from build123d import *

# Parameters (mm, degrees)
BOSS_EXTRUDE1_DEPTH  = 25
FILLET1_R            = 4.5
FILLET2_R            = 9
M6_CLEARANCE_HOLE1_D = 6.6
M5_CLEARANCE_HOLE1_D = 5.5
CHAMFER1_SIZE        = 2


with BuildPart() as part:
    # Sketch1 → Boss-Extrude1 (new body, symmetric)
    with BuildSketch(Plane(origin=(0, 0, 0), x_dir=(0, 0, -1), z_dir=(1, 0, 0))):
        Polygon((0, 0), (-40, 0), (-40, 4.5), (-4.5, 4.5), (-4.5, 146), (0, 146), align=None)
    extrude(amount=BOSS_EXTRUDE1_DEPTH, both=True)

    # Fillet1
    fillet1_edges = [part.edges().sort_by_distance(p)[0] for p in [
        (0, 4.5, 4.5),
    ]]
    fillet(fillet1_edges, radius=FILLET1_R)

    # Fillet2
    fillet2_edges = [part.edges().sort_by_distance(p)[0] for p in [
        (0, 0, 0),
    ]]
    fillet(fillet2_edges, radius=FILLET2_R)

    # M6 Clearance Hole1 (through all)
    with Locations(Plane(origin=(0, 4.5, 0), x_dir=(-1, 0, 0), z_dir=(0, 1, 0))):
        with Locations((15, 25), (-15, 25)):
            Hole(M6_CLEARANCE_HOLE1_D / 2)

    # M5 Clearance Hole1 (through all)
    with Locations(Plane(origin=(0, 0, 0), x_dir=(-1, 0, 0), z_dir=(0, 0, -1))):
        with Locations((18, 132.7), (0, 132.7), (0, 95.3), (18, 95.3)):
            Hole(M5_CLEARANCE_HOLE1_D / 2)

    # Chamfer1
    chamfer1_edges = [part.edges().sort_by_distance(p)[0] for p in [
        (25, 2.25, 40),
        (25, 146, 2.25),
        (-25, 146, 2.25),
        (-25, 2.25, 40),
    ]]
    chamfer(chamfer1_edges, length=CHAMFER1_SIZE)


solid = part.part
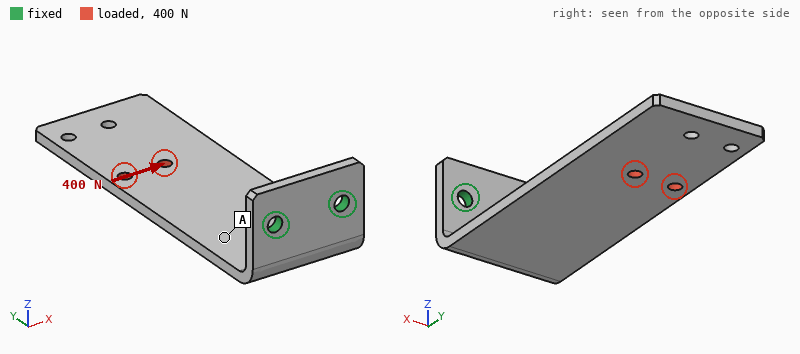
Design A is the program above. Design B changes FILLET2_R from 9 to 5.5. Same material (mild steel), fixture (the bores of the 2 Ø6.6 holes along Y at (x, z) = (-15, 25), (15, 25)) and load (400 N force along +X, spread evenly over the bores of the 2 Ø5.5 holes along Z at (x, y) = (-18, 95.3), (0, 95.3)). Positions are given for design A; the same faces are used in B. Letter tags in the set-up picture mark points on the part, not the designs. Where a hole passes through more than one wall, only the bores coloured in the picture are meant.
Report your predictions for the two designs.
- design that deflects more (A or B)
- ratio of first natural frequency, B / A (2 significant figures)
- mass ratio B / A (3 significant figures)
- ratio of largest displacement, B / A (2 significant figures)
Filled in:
A
1.0
1.01
0.90
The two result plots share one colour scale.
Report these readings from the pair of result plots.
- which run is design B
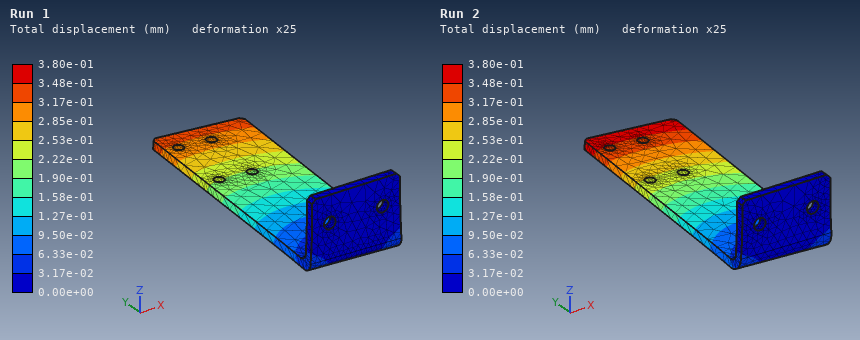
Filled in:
Run 1
